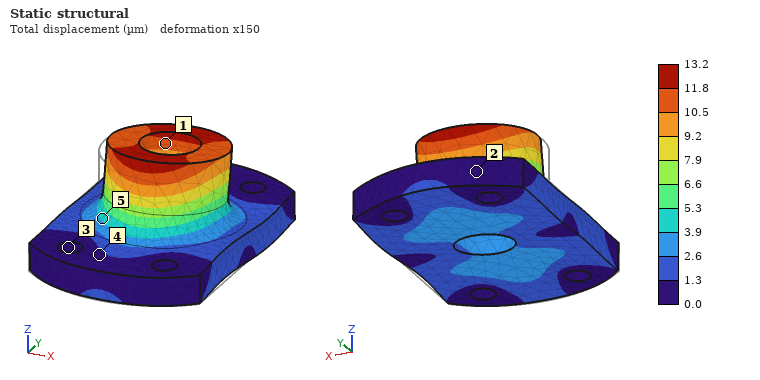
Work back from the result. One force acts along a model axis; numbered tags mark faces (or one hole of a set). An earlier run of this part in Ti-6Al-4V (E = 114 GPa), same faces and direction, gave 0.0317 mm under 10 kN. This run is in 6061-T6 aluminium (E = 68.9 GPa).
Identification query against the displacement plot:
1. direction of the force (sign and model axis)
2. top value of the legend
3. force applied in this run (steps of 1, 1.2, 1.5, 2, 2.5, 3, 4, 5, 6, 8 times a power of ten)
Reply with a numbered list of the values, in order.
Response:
1. +Y
2. 13.2 µm
3. 2.5 kN
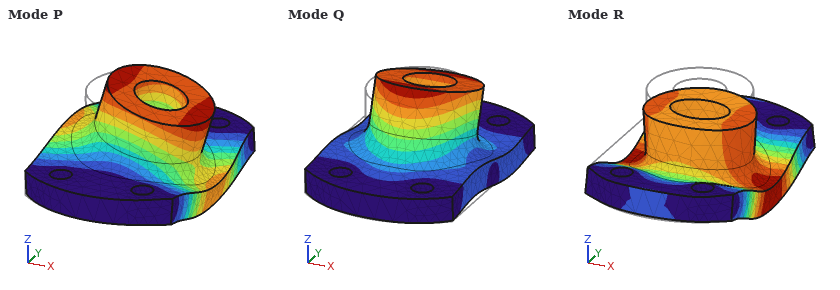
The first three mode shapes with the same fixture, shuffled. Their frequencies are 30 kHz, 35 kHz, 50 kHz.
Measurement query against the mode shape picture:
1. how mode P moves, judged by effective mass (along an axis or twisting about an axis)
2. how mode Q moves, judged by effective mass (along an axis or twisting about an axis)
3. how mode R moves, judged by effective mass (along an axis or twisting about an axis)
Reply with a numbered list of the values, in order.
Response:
1. along X
2. along Y
3. along Z
